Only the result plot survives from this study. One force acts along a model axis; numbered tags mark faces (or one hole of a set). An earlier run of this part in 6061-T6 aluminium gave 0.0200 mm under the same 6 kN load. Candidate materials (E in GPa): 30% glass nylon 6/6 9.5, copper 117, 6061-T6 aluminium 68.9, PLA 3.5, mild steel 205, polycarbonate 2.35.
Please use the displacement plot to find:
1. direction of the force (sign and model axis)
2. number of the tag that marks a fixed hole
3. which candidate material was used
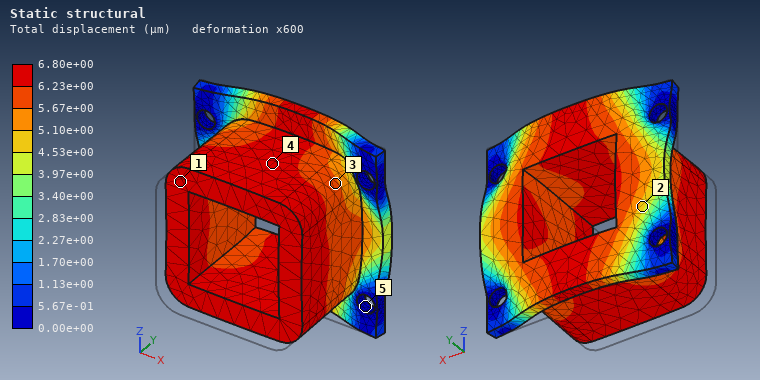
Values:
+Y
5
mild steel
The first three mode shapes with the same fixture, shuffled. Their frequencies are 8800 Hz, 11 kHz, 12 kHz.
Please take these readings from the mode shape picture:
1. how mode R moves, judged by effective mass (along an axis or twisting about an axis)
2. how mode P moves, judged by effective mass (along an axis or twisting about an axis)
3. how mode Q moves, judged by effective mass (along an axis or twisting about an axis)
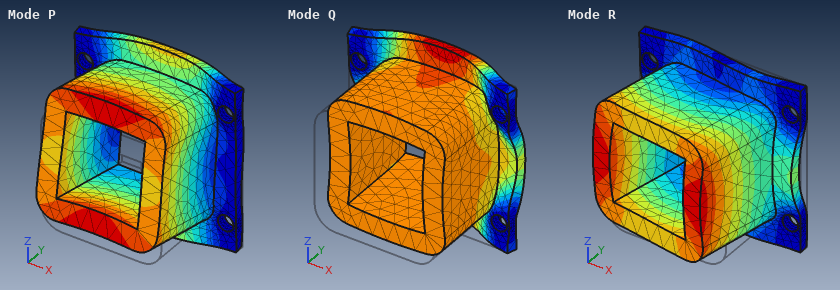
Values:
along X
along Z
along Y
